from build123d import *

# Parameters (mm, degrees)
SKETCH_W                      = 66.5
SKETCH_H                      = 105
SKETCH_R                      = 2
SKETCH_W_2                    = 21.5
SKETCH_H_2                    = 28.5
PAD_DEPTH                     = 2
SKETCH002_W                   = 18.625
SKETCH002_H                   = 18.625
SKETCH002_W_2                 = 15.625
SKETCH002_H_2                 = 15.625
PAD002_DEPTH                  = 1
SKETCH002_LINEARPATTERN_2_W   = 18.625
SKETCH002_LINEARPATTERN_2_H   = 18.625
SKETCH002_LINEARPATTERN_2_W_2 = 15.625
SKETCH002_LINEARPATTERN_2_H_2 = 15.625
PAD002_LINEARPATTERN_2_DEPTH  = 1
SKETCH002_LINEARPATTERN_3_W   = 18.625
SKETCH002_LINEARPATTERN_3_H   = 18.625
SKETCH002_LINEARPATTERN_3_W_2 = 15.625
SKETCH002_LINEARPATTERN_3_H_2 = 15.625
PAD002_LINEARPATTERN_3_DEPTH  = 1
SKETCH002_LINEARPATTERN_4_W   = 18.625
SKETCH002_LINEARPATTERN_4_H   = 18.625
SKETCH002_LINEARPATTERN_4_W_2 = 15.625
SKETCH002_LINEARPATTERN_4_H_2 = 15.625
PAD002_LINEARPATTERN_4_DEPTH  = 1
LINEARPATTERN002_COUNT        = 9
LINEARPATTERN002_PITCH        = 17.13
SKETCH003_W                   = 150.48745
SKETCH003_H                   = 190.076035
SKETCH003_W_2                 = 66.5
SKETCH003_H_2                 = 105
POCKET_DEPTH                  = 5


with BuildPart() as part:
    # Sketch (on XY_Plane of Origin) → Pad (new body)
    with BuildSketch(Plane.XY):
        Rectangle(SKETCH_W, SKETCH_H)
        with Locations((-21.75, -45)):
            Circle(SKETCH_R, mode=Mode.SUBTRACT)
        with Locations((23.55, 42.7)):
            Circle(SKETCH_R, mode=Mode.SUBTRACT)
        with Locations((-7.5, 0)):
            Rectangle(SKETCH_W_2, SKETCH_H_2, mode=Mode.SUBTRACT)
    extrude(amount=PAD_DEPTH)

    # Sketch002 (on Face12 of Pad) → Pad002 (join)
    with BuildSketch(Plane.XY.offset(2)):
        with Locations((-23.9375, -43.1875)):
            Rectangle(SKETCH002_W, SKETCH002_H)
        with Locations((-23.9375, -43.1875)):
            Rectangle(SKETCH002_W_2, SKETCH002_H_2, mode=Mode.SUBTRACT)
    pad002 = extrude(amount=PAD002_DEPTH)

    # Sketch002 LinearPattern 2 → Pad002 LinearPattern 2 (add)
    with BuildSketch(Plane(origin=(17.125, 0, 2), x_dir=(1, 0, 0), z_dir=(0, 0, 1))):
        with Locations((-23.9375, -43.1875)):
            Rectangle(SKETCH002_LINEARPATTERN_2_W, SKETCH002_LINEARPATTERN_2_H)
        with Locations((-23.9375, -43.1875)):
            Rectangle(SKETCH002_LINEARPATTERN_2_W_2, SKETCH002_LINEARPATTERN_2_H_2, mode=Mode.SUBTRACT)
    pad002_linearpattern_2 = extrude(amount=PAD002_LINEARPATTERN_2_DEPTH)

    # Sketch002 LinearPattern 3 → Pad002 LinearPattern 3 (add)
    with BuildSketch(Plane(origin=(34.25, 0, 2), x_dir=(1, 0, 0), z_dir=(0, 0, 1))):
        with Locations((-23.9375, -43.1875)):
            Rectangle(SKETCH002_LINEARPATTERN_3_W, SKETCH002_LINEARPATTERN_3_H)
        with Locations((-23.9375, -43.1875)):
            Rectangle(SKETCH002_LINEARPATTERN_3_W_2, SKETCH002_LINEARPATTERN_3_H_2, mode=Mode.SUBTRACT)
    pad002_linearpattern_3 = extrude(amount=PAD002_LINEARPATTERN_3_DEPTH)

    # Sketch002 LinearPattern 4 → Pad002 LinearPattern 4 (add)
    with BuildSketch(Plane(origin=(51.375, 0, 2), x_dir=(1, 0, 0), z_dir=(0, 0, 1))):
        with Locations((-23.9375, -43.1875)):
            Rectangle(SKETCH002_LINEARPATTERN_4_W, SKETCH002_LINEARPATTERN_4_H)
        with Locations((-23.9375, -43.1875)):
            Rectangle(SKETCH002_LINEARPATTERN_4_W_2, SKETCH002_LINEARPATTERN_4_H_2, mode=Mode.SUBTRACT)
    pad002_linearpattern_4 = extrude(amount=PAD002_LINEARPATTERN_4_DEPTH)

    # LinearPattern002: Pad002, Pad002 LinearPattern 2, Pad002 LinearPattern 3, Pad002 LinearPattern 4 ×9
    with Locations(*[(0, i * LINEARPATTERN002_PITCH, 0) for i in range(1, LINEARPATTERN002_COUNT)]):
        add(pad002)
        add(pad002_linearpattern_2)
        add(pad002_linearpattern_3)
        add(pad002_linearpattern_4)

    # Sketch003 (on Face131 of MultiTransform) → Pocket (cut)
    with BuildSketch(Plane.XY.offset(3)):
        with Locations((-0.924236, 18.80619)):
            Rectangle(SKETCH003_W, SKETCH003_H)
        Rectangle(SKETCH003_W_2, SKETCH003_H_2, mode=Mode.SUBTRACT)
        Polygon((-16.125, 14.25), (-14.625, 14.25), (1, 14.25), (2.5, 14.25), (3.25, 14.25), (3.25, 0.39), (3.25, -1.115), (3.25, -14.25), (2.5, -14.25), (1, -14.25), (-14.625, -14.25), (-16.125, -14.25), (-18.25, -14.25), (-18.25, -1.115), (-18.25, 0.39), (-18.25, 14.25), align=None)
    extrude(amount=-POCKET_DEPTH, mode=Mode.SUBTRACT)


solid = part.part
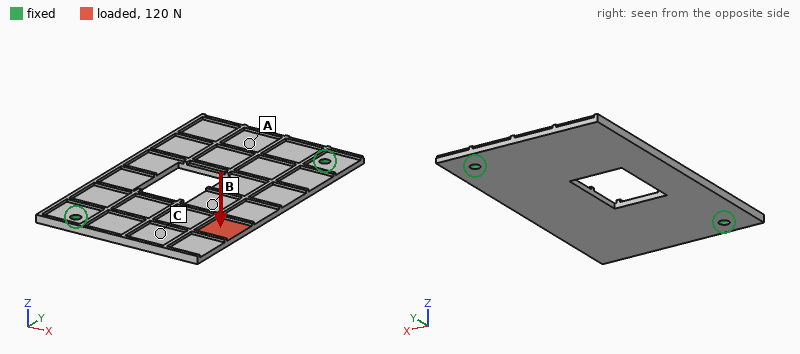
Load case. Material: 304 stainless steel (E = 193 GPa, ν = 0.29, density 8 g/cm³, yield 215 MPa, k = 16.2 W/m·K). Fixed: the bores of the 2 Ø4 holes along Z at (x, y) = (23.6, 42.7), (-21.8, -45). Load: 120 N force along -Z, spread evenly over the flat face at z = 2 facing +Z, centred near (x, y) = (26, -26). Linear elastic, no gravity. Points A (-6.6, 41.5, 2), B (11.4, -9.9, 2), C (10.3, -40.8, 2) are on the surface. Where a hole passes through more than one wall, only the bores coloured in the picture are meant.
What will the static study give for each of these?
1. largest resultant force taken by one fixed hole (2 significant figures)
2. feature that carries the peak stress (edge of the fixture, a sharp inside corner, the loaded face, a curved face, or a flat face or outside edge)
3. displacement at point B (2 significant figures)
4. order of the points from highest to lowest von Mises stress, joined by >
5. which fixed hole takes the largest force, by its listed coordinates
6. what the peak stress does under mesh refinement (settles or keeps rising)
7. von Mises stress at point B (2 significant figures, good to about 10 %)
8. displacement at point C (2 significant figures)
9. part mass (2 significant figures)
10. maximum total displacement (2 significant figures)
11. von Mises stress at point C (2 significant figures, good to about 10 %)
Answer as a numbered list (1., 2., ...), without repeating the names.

1. 77 N
2. edge of the fixture
3. 0.19 mm
4. B > C > A
5. (-21.8, -45)
6. keeps rising
7. 47 MPa
8. 0.24 mm
9. 110 g
10. 0.51 mm
11. 26 MPa
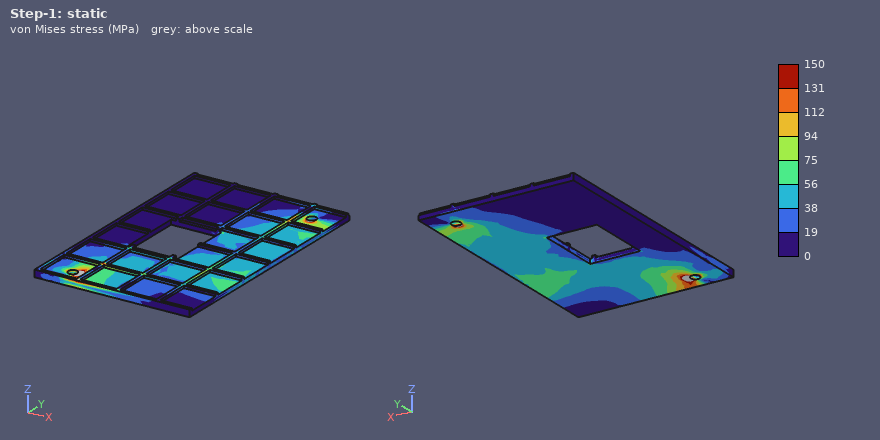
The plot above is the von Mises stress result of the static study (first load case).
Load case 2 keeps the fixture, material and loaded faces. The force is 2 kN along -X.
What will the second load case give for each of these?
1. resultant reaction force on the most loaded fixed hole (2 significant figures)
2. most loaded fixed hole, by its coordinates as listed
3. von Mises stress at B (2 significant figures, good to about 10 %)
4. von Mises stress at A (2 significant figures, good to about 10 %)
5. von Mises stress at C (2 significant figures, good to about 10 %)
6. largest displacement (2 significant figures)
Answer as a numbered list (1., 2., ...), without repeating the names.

1. 1.7 kN
2. (-21.8, -45)
3. 27 MPa
4. 8.5 MPa
5. 52 MPa
6. 0.24 mm
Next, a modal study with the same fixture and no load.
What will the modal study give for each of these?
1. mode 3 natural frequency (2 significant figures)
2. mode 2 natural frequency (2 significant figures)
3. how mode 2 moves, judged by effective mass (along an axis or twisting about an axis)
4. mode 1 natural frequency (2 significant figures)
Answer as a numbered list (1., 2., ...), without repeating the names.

1. 1300 Hz
2. 680 Hz
3. along Z
4. 560 Hz
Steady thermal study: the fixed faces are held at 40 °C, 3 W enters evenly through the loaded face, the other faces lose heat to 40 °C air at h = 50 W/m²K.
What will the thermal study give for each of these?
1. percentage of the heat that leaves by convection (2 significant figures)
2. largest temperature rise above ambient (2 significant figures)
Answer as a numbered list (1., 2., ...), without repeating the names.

1. 95 %
2. 35 K
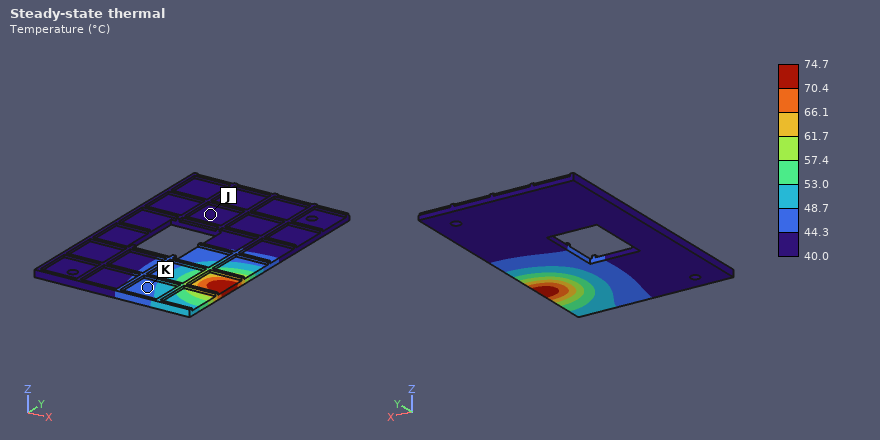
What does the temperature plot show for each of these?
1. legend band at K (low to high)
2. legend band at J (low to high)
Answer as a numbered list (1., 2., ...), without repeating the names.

1. 44.3 to 48.7 °C
2. 40.0 to 44.3 °C
